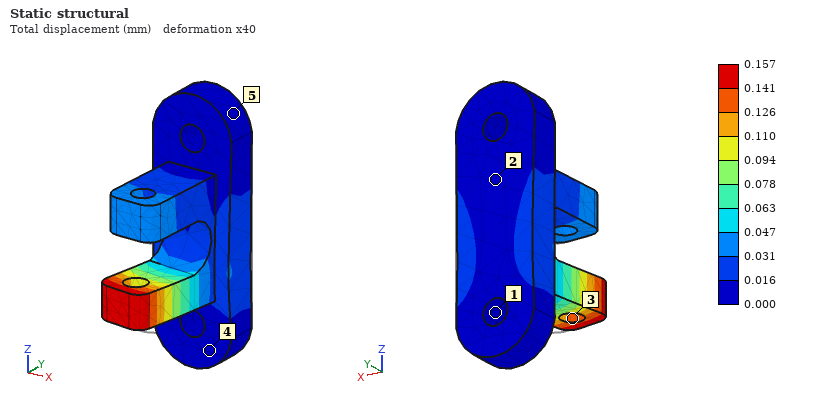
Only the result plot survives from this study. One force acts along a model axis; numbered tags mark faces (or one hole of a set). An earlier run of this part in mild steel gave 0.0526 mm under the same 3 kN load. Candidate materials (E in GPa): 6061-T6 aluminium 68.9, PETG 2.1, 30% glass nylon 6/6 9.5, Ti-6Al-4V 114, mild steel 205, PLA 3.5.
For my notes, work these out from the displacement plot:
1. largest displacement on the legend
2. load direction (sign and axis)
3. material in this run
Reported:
0.157 mm
-X
6061-T6 aluminium
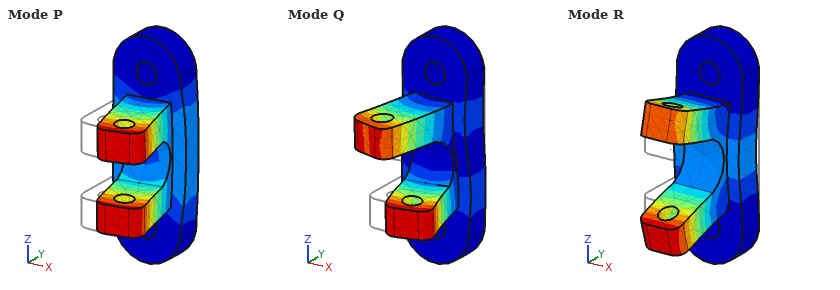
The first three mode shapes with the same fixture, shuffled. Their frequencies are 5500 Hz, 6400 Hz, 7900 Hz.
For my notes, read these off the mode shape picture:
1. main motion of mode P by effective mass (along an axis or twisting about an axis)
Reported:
along X
